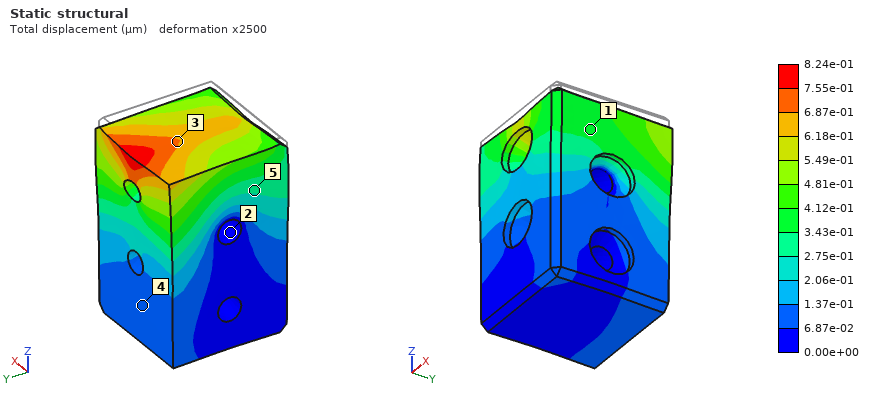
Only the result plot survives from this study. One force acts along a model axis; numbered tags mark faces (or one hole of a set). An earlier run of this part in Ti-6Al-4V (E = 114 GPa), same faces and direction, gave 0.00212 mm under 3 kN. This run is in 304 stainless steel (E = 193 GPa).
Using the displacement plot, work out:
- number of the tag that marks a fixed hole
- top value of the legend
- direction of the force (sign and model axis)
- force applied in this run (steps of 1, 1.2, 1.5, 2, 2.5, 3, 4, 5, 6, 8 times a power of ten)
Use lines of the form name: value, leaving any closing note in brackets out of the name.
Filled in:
number of the tag that marks a fixed hole: 2
top value of the legend: 8.24e-01 µm
direction of the force: -Z
force applied in this run: 2 kN
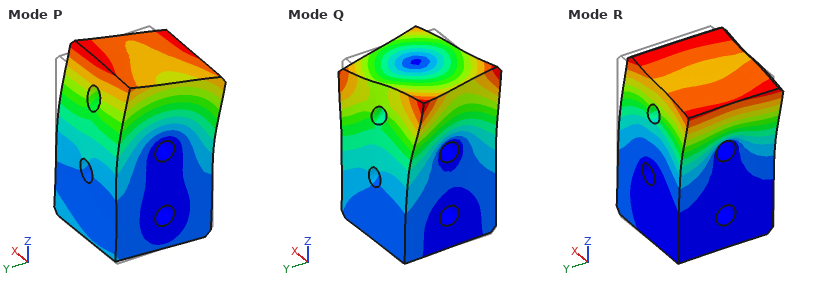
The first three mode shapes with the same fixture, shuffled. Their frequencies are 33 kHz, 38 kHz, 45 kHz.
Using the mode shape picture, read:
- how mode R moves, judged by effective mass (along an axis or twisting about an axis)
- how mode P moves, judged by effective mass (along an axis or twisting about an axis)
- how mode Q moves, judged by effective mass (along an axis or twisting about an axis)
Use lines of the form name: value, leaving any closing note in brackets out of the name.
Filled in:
how mode R moves, judged by effective mass: along X
how mode P moves, judged by effective mass: along Y
how mode Q moves, judged by effective mass: twisting about Z
